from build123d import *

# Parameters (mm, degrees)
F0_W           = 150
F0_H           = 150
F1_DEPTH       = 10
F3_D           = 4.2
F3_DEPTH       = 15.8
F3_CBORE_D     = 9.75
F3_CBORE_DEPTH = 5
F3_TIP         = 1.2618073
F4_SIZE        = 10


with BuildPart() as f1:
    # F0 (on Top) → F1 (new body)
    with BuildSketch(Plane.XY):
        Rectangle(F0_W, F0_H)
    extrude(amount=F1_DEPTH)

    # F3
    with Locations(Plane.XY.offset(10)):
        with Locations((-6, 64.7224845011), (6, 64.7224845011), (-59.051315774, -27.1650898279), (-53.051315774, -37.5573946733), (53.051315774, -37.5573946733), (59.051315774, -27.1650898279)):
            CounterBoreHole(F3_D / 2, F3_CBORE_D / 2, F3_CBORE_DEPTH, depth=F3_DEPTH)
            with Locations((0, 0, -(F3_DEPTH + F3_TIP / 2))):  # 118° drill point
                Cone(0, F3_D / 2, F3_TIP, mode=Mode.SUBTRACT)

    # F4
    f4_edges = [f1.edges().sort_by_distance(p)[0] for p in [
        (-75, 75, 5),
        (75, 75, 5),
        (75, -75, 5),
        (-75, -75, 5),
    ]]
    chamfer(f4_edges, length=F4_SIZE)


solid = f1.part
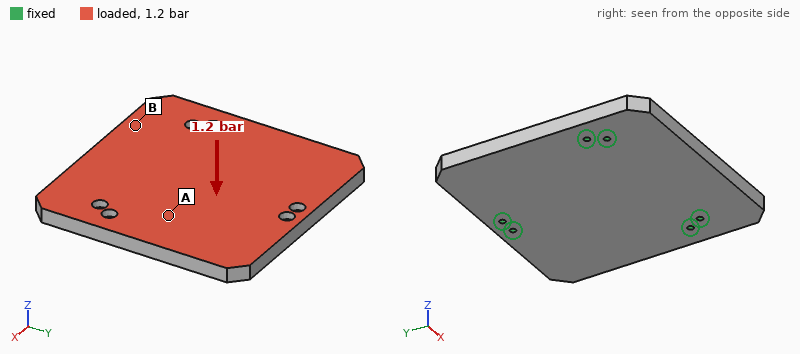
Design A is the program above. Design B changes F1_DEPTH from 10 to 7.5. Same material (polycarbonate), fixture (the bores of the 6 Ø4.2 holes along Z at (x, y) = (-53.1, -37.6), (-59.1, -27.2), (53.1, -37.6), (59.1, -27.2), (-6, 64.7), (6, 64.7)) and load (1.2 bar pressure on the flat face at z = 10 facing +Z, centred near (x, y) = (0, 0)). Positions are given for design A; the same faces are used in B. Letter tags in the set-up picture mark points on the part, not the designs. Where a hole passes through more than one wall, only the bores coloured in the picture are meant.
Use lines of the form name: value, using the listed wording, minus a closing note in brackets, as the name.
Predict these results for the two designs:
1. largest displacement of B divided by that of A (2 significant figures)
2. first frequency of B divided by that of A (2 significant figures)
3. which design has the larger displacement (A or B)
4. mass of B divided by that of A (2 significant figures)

largest displacement of B divided by that of A: 2.2
first frequency of B divided by that of A: 0.83
which design has the larger displacement: B
mass of B divided by that of A: 0.75
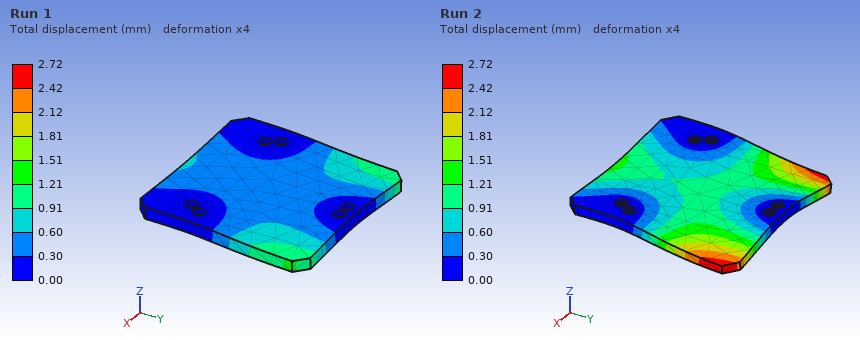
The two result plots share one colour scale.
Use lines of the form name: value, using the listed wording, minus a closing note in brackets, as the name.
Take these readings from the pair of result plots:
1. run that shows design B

run that shows design B: Run 2
